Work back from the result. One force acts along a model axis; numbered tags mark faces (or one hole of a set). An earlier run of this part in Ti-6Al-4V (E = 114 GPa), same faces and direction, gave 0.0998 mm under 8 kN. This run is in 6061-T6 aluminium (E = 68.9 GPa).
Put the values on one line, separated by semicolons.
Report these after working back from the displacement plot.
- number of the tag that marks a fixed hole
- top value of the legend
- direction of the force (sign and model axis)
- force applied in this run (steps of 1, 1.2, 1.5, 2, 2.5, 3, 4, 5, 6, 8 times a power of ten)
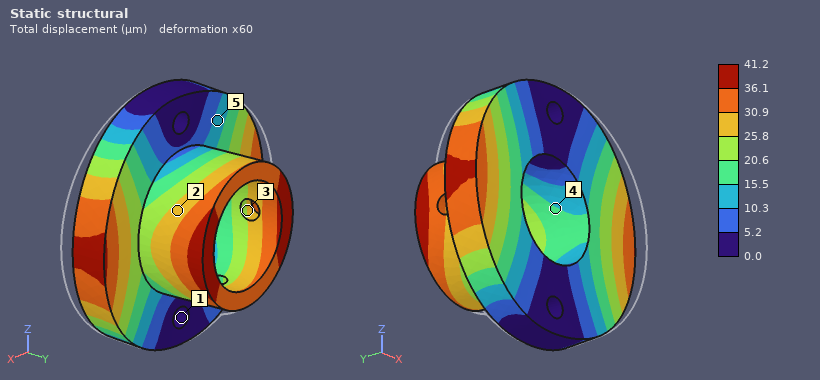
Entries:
1; 41.2 µm; -X; 2 kN
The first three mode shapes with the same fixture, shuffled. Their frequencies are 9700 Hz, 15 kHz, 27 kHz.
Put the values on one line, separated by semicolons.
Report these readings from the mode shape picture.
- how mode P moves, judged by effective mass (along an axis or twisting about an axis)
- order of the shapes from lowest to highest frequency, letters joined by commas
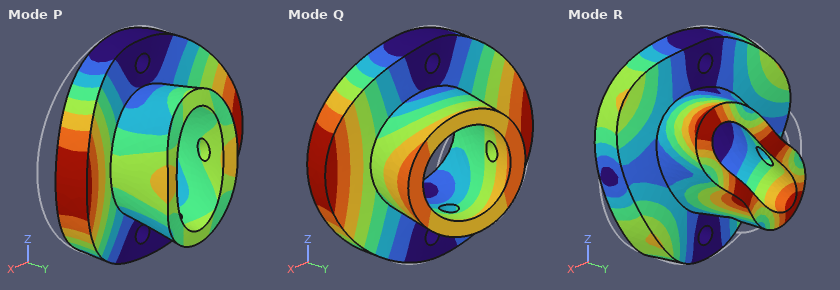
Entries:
along Y; Q, P, R
